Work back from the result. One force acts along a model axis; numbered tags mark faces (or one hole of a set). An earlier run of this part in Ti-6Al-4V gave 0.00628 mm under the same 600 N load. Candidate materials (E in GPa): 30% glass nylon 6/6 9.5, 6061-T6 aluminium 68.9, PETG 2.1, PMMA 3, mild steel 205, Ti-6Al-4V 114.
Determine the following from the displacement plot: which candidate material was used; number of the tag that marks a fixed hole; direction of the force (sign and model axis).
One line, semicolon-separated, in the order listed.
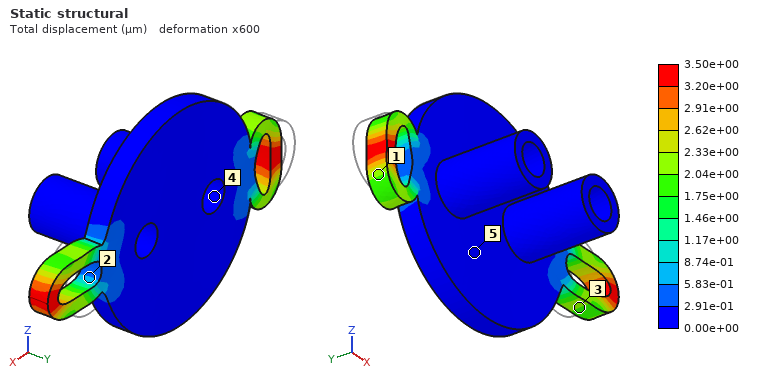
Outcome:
mild steel; 4; +X
